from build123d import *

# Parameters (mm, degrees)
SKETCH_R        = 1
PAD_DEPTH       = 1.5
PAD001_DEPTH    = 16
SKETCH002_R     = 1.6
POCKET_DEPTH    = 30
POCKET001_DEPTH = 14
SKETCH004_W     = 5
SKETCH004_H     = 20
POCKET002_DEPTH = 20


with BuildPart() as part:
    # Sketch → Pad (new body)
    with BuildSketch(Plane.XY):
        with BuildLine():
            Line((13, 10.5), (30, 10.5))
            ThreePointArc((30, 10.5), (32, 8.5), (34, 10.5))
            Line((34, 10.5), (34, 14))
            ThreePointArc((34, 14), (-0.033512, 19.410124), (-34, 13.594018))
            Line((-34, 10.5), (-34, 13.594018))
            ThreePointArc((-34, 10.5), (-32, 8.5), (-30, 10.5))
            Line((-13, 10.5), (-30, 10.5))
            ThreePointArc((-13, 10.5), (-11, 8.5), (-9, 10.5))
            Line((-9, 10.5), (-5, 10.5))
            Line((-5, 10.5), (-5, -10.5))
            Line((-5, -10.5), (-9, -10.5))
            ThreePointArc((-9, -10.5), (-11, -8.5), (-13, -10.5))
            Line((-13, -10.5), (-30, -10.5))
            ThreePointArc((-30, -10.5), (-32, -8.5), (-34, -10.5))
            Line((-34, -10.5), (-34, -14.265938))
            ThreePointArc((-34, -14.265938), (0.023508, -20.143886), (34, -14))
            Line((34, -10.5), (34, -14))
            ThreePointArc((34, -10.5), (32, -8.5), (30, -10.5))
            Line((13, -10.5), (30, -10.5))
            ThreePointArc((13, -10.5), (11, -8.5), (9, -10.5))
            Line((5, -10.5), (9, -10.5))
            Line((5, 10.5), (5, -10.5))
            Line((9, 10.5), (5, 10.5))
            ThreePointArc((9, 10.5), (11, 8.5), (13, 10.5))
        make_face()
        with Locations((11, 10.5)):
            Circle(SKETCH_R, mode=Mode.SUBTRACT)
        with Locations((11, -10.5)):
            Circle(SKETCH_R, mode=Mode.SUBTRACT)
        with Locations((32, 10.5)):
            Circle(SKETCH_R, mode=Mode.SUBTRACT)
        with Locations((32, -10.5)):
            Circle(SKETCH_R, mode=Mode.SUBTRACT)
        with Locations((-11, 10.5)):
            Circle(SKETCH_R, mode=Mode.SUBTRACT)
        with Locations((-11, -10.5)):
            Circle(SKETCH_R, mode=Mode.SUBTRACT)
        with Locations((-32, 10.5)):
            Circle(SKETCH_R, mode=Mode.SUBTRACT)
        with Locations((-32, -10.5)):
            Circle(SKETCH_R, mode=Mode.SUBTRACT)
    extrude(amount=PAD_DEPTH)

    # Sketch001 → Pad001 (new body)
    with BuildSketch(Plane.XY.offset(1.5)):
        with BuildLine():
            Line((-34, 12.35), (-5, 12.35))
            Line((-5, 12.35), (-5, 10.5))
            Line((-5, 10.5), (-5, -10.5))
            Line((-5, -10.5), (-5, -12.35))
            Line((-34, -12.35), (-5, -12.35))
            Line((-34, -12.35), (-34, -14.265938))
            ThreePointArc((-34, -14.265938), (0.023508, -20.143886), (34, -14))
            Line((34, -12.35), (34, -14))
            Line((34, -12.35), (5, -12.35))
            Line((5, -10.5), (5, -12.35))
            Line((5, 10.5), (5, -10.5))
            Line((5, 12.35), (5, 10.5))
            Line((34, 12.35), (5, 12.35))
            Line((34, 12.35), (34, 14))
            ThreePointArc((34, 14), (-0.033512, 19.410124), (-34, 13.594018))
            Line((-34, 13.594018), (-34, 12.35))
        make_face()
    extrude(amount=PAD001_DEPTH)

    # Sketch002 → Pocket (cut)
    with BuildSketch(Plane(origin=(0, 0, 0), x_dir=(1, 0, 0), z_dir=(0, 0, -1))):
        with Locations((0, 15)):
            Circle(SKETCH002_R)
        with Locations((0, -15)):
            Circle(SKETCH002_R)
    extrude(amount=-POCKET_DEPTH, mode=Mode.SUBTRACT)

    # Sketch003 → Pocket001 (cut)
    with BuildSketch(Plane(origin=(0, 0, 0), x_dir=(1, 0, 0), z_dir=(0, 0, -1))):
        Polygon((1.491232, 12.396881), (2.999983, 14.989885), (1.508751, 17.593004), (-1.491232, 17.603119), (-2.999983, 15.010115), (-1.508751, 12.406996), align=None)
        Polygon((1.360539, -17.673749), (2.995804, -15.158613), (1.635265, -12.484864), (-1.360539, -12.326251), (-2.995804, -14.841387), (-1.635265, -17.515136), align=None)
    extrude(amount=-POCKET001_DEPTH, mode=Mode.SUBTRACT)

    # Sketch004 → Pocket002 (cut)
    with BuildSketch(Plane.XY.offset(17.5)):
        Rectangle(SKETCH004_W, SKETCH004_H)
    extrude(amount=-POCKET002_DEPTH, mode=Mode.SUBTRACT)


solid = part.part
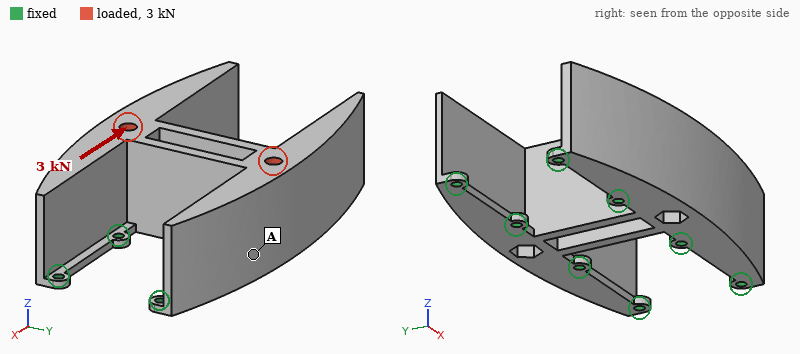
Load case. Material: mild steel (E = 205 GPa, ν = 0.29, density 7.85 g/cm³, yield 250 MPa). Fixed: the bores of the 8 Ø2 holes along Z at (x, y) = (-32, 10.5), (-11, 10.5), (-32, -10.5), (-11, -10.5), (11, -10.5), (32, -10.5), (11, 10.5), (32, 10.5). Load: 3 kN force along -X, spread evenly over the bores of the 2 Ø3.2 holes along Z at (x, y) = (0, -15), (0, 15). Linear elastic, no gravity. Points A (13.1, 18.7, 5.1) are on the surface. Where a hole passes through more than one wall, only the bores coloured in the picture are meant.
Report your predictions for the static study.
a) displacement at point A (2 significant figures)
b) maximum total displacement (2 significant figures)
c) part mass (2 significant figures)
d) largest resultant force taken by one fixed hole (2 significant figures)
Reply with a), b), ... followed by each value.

a) 2.8 µm
b) 7.2 µm
c) 120 g
d) 490 N
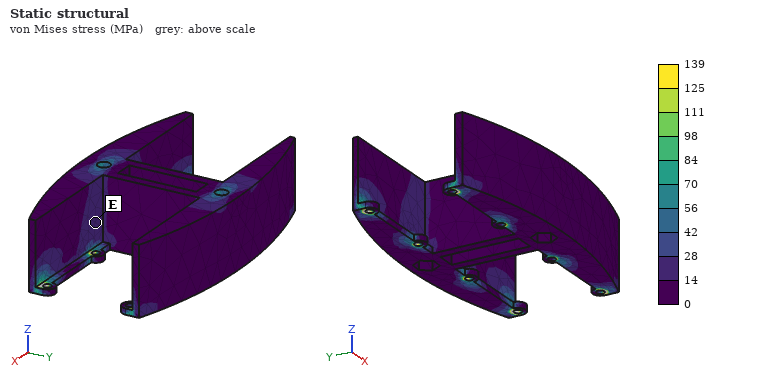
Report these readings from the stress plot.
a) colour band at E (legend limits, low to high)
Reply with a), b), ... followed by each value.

a) 14 to 28 MPa
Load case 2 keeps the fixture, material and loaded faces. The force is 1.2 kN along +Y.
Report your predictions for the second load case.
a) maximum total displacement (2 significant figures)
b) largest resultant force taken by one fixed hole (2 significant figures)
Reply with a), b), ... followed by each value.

a) 14 µm
b) 440 N
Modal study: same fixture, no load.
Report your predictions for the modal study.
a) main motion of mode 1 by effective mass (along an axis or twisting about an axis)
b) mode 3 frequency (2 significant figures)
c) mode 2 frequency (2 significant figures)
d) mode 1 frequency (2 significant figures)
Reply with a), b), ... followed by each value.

a) along Y
b) 10 kHz
c) 9700 Hz
d) 6000 Hz
